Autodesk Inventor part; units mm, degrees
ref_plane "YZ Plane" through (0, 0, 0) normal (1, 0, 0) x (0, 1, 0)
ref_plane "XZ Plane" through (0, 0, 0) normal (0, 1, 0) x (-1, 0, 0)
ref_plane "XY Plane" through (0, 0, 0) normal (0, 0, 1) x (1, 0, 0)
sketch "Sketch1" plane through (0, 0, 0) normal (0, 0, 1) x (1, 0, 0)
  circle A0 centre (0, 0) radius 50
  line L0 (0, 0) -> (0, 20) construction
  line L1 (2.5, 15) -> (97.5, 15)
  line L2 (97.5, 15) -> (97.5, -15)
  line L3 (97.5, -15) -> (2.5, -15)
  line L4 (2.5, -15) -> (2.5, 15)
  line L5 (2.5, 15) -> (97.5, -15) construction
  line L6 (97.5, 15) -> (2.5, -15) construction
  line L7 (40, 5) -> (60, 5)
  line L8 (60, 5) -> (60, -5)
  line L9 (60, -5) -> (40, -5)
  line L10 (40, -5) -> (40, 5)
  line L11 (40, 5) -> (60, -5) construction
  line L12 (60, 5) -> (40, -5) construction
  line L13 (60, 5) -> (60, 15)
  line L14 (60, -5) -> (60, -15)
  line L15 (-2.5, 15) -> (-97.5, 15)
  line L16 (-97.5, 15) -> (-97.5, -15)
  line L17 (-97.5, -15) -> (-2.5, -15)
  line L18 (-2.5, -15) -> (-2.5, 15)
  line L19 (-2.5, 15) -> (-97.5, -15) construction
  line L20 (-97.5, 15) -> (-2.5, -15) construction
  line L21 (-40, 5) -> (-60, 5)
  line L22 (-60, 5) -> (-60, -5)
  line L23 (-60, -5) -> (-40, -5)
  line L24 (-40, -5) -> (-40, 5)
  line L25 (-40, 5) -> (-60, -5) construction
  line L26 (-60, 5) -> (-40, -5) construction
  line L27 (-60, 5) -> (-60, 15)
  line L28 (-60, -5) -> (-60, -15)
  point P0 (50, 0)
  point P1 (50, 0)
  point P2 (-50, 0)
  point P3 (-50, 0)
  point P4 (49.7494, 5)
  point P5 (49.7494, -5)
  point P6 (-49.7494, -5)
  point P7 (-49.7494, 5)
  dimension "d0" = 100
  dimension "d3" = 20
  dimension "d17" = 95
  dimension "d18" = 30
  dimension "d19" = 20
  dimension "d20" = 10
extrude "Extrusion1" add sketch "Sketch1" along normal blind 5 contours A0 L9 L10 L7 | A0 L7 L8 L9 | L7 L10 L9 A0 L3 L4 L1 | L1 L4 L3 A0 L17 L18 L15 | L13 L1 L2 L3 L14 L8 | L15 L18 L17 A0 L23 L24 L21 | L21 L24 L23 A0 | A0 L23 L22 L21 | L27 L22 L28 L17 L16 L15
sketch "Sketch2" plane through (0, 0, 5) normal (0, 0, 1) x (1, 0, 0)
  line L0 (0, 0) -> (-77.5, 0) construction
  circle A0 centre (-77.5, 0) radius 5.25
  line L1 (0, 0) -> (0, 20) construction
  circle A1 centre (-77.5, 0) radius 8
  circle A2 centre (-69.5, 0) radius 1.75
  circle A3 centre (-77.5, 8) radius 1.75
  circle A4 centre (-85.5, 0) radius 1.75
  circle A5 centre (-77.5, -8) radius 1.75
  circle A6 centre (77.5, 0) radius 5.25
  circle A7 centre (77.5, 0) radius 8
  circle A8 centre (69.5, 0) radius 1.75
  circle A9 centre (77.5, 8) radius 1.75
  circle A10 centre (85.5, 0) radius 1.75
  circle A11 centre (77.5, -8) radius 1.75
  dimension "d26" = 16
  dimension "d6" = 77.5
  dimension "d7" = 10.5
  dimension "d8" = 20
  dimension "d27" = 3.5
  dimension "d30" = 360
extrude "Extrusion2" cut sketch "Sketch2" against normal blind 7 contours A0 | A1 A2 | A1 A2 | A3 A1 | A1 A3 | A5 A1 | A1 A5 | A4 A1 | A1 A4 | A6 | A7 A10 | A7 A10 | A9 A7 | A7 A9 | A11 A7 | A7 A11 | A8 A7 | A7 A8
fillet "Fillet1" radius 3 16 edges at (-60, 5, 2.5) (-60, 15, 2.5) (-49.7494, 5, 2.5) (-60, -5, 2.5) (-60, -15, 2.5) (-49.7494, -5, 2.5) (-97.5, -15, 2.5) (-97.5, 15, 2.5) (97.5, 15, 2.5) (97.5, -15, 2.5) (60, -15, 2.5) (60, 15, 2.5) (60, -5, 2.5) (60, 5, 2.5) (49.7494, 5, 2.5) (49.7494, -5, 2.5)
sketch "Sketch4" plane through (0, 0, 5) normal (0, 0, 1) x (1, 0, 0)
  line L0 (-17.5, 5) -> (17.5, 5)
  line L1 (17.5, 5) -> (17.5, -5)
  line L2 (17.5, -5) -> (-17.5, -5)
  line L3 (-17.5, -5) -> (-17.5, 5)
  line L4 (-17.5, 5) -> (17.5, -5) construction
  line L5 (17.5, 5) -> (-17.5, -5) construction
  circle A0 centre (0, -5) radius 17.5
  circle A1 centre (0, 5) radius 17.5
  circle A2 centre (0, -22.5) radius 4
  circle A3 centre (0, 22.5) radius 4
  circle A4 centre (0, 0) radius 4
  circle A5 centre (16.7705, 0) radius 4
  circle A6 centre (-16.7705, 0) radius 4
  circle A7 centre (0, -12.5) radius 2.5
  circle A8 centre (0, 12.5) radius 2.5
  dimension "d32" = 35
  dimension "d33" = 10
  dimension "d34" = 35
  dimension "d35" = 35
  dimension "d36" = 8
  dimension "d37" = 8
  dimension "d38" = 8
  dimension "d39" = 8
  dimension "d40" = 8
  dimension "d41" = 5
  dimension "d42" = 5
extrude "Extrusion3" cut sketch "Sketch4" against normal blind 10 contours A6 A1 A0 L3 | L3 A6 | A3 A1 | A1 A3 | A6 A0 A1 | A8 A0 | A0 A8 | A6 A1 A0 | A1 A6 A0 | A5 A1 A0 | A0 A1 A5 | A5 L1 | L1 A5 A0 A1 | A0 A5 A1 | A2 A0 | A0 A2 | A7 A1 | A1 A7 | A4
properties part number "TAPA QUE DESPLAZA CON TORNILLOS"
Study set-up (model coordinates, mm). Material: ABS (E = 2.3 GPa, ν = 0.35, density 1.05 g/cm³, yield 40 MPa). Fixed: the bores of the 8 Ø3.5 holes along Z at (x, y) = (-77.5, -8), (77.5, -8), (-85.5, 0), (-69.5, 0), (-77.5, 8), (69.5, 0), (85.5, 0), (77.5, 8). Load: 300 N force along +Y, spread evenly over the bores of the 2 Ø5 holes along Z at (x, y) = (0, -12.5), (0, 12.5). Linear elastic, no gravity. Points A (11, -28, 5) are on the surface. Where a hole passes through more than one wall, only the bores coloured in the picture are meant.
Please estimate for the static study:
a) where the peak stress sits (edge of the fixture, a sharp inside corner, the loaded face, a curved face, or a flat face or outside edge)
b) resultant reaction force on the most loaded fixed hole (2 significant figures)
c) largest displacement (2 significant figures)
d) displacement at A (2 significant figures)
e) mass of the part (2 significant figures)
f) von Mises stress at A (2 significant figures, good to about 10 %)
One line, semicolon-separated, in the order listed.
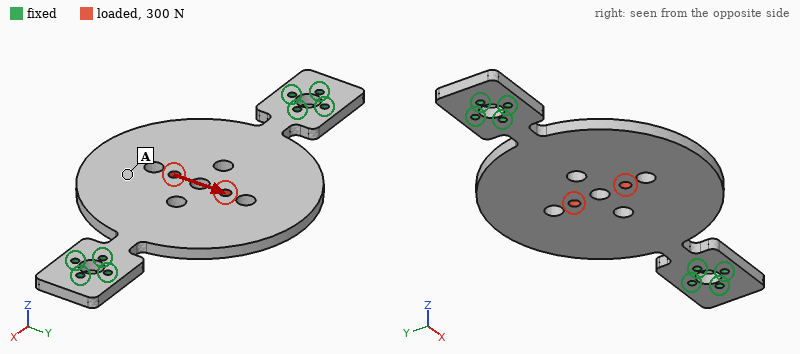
a curved face; 150 N; 0.16 mm; 0.15 mm; 51 g; 1.2 MPa
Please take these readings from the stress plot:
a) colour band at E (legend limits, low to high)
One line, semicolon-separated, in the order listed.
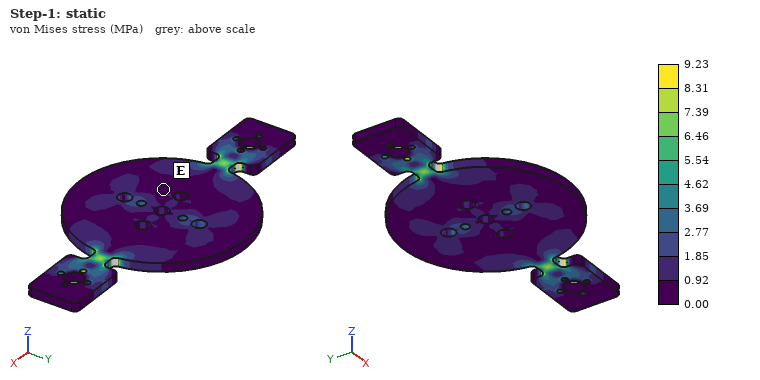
0.00 to 0.92 MPa
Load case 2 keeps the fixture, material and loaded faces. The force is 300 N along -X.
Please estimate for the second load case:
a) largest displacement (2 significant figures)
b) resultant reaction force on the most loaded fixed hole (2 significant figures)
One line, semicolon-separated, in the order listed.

48 µm; 92 N
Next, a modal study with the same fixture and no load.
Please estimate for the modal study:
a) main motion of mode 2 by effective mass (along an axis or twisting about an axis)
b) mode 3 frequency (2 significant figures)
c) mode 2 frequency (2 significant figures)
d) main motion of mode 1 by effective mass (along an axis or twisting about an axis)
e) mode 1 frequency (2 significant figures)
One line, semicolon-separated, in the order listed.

along Z; 700 Hz; 230 Hz; twisting about X; 160 Hz
